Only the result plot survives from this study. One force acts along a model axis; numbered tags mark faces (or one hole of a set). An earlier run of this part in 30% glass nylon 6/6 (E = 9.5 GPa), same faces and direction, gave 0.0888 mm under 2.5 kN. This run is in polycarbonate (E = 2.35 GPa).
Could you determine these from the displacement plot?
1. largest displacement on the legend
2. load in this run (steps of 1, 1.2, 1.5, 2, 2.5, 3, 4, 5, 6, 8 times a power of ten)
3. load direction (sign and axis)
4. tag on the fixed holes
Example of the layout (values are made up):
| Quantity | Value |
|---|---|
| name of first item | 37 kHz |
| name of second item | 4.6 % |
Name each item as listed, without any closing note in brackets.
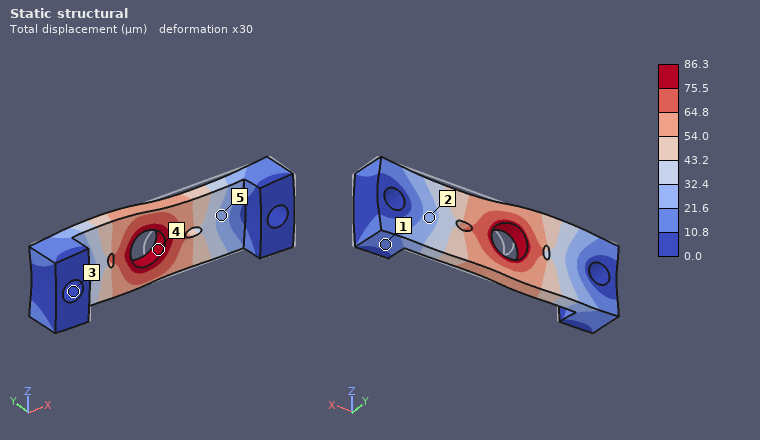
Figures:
| Quantity | Value |
|---|---|
| largest displacement on the legend | 86.3 µm |
| load in this run | 600 N |
| load direction | -X |
| tag on the fixed holes | 3 |
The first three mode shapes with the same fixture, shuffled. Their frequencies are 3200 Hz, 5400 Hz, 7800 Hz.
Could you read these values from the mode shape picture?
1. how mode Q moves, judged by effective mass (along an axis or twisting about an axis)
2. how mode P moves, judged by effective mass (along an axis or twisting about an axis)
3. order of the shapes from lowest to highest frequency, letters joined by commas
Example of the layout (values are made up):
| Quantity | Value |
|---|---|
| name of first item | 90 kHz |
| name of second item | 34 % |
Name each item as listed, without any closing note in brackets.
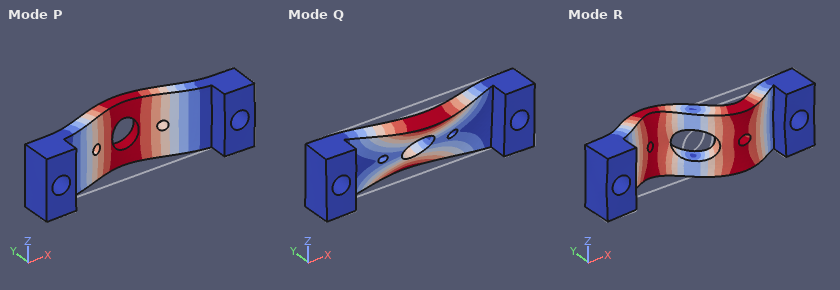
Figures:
| Quantity | Value |
|---|---|
| how mode Q moves, judged by effective mass | twisting about X |
| how mode P moves, judged by effective mass | along Y |
| order of the shapes from lowest to highest frequency, letters joined by commas | P, Q, R |
